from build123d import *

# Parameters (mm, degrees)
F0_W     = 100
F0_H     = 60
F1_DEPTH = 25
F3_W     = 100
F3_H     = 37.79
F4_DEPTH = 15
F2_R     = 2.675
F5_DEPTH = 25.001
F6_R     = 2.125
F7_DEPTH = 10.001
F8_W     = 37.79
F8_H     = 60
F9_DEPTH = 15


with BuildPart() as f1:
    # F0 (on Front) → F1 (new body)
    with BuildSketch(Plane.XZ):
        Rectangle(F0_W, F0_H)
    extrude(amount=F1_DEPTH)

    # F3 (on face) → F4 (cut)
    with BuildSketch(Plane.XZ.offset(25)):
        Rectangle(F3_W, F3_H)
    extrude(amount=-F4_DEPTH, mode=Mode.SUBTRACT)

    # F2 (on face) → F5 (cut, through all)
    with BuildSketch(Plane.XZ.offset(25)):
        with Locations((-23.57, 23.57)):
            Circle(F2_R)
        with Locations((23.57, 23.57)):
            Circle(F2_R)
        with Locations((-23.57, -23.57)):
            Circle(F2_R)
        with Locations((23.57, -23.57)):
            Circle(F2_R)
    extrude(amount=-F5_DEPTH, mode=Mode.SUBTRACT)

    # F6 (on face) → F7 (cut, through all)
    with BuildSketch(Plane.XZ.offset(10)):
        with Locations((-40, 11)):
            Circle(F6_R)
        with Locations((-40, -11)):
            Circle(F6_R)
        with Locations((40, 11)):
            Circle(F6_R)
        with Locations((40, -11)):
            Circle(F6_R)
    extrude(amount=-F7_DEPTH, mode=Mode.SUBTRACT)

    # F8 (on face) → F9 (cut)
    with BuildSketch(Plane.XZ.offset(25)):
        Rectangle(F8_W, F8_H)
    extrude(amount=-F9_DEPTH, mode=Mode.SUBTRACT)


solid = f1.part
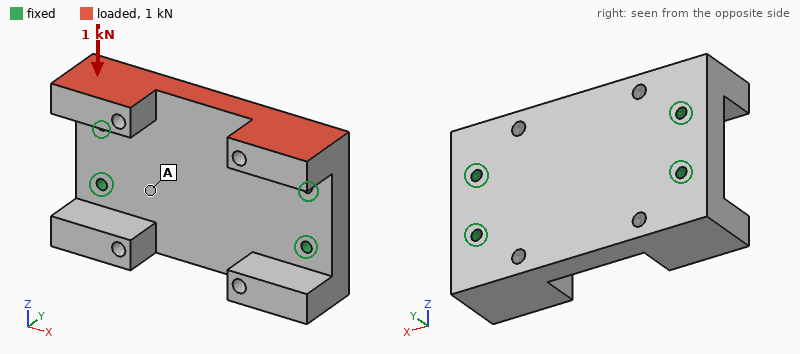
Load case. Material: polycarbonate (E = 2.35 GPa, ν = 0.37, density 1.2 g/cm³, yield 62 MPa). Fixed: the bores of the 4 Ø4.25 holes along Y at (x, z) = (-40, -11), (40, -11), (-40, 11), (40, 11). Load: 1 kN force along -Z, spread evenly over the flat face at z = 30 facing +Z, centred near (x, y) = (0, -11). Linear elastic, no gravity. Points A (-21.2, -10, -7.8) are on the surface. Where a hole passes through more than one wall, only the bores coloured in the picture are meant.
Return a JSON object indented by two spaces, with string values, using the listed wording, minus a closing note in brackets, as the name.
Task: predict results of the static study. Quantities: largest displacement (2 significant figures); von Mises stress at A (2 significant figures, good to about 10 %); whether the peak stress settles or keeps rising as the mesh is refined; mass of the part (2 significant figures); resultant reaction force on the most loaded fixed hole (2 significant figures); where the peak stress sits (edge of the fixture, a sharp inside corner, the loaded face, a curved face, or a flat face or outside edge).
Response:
{
  "largest displacement": "0.20 mm",
  "von Mises stress at A": "1.2 MPa",
  "whether the peak stress settles or keeps rising as the mesh is refined": "keeps rising",
  "mass of the part": "93 g",
  "resultant reaction force on the most loaded fixed hole": "350 N",
  "where the peak stress sits": "edge of the fixture"
}
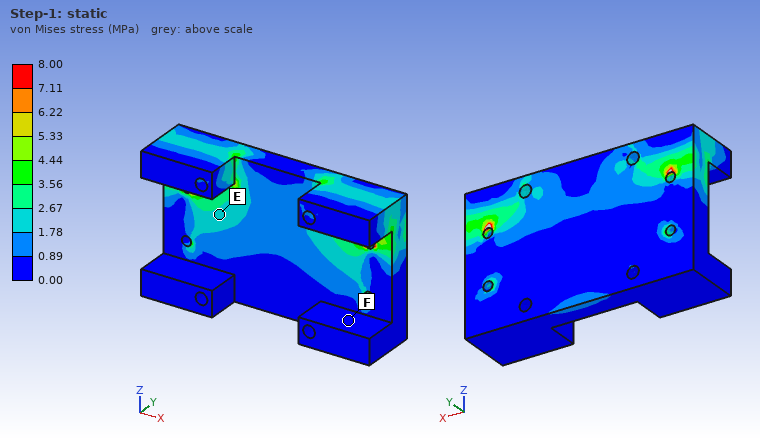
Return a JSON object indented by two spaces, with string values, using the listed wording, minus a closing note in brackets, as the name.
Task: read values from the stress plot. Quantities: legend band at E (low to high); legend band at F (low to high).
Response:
{
  "legend band at E": "1.78 to 2.67 MPa",
  "legend band at F": "0.00 to 0.89 MPa"
}
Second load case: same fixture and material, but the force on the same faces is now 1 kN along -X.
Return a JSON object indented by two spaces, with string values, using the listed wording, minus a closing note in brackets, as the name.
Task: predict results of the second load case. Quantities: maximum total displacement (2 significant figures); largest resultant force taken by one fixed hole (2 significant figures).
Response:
{
  "maximum total displacement": "96 µm",
  "largest resultant force taken by one fixed hole": "460 N"
}
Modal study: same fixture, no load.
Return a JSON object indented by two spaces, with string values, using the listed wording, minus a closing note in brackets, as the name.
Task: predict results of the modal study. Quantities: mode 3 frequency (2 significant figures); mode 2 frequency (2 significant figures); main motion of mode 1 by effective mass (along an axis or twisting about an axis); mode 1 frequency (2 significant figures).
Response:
{
  "mode 3 frequency": "2500 Hz",
  "mode 2 frequency": "1700 Hz",
  "main motion of mode 1 by effective mass": "along Y",
  "mode 1 frequency": "1600 Hz"
}
